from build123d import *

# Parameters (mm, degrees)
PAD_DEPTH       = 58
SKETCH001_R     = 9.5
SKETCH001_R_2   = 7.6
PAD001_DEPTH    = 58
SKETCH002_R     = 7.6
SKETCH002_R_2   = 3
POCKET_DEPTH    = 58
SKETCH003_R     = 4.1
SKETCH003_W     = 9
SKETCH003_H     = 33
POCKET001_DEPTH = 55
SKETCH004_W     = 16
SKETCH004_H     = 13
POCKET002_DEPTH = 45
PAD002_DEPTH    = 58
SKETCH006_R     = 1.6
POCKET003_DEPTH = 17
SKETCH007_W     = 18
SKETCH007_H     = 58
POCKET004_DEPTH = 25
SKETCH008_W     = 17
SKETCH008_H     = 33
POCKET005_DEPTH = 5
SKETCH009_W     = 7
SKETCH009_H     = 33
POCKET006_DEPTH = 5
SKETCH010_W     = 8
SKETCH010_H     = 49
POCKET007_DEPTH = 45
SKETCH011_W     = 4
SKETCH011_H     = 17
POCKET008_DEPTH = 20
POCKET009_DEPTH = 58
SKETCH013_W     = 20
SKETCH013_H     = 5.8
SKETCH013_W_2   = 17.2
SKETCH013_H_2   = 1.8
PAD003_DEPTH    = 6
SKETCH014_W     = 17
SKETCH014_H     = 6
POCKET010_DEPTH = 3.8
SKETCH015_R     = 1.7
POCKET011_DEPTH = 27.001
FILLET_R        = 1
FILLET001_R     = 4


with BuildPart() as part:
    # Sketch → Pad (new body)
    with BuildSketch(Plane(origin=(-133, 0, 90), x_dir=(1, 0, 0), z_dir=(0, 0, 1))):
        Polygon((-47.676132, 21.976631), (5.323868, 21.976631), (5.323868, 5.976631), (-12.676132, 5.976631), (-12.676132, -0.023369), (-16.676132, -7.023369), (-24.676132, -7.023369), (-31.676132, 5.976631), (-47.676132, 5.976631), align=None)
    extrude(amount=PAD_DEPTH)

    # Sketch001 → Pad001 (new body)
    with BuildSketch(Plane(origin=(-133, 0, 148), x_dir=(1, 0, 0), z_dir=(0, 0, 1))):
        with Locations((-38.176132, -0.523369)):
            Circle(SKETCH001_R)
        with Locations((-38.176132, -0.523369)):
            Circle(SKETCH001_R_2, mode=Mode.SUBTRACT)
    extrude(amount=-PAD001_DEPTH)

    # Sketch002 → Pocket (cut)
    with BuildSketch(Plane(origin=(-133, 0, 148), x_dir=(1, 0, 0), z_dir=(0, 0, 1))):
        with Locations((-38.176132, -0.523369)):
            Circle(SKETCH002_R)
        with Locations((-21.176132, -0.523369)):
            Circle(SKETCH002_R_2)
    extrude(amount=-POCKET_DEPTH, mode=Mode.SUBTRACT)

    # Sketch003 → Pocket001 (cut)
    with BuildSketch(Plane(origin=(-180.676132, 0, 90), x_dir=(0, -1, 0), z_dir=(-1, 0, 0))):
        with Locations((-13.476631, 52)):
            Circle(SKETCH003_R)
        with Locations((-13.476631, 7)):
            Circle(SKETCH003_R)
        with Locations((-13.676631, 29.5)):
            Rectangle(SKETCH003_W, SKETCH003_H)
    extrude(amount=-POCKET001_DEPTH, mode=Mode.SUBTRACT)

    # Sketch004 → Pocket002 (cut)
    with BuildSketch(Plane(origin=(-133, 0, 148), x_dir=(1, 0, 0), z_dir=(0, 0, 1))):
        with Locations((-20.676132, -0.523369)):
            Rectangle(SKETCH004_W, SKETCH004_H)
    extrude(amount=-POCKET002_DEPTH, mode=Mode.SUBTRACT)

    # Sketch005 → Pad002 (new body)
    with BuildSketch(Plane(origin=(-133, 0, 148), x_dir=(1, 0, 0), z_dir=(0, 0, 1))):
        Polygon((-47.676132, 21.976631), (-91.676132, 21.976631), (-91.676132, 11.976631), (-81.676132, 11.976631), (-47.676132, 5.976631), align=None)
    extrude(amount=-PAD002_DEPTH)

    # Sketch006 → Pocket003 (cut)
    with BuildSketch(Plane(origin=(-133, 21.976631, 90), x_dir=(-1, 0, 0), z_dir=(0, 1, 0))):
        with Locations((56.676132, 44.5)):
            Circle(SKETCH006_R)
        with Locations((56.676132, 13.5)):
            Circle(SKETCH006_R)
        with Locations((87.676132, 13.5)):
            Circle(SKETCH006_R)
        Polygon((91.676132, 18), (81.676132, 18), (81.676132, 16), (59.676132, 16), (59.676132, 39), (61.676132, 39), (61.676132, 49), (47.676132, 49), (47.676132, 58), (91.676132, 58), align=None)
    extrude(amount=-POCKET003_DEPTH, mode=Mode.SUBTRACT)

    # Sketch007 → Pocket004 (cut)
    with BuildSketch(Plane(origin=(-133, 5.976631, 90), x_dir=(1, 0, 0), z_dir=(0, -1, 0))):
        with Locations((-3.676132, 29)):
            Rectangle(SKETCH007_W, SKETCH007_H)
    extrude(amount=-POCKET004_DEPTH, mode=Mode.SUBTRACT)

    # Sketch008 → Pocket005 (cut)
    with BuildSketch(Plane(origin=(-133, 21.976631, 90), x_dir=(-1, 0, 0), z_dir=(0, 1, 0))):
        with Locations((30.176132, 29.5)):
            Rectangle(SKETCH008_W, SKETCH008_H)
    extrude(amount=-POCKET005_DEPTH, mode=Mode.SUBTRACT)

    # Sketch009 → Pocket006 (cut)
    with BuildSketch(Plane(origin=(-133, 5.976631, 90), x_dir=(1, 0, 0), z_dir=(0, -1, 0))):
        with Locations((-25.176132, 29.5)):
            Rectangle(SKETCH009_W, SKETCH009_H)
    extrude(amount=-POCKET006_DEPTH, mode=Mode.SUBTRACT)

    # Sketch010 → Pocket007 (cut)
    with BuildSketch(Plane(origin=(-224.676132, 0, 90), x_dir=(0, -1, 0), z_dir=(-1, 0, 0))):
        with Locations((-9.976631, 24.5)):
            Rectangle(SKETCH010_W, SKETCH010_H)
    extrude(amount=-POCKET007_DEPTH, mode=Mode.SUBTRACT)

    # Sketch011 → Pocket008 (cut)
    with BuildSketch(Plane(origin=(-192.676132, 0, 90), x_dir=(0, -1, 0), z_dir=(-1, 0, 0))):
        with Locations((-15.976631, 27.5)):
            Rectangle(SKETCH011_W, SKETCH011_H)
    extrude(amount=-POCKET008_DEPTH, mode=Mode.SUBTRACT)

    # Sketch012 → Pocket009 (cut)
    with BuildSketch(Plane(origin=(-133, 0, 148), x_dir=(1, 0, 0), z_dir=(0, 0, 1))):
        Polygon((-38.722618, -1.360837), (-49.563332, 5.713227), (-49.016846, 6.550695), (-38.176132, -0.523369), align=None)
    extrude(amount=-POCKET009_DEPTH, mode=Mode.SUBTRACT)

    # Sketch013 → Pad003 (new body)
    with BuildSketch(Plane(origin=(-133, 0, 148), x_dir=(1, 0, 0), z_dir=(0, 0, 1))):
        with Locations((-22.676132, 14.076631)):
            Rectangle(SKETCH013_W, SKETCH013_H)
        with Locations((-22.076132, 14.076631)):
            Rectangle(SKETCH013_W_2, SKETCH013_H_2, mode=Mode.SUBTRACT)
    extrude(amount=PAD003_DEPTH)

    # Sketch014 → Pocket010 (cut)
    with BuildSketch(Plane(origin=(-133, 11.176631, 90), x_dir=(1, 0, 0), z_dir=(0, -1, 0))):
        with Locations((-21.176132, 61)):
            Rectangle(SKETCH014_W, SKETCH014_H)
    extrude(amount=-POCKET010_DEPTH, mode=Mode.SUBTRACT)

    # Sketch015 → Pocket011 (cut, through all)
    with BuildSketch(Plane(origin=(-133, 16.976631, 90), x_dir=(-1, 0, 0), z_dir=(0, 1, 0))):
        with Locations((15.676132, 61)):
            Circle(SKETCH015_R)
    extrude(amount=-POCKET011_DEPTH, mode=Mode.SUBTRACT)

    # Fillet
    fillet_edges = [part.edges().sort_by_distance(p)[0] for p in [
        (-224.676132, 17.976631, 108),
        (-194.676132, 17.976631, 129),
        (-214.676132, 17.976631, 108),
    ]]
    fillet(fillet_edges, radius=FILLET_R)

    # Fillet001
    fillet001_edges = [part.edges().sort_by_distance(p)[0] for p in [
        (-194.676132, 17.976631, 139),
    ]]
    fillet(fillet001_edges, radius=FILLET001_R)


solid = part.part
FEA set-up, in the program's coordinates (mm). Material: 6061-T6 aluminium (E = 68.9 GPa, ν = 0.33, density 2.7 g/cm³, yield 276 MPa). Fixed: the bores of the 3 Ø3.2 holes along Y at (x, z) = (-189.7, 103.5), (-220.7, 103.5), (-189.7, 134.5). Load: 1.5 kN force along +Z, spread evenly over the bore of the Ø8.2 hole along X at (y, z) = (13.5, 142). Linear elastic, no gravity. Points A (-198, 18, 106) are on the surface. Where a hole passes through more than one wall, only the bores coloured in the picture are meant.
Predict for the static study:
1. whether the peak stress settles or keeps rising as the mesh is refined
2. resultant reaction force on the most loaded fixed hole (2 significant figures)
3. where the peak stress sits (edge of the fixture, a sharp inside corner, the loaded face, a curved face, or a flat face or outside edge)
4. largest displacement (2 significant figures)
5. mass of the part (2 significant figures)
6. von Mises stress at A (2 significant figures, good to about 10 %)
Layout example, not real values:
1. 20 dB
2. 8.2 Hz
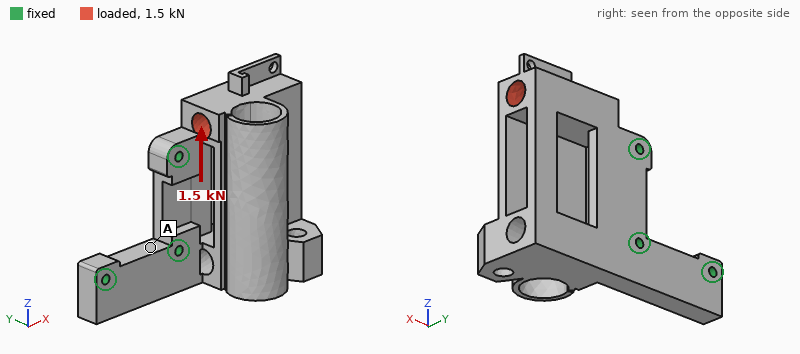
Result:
1. keeps rising
2. 1.2 kN
3. a sharp inside corner
4. 52 µm
5. 81 g
6. 5.4 MPa
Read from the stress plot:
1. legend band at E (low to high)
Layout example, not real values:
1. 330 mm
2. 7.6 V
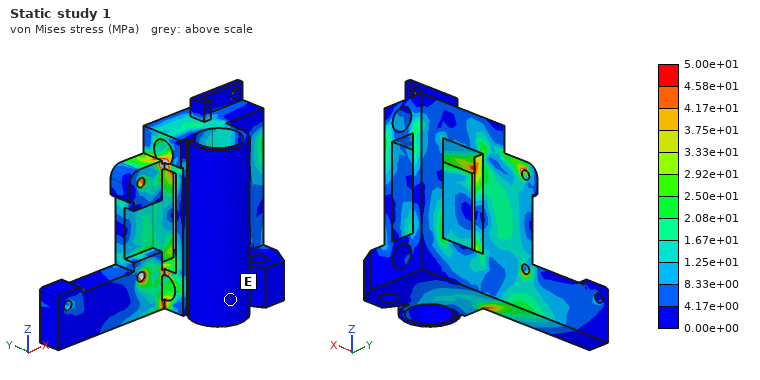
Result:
1. 0.00e+00 to 4.17e+00 MPa
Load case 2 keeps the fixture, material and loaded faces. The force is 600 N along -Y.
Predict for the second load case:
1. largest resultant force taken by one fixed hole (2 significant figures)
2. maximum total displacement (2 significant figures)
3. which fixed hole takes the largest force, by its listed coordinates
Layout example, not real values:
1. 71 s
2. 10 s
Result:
1. 600 N
2. 0.21 mm
3. (-189.7, 134.5)
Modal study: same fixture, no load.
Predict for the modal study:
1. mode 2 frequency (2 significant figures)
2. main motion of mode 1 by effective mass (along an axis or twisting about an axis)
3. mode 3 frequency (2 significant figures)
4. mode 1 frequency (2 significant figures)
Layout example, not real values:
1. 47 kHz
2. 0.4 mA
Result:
1. 1900 Hz
2. along Y
3. 2400 Hz
4. 1600 Hz
